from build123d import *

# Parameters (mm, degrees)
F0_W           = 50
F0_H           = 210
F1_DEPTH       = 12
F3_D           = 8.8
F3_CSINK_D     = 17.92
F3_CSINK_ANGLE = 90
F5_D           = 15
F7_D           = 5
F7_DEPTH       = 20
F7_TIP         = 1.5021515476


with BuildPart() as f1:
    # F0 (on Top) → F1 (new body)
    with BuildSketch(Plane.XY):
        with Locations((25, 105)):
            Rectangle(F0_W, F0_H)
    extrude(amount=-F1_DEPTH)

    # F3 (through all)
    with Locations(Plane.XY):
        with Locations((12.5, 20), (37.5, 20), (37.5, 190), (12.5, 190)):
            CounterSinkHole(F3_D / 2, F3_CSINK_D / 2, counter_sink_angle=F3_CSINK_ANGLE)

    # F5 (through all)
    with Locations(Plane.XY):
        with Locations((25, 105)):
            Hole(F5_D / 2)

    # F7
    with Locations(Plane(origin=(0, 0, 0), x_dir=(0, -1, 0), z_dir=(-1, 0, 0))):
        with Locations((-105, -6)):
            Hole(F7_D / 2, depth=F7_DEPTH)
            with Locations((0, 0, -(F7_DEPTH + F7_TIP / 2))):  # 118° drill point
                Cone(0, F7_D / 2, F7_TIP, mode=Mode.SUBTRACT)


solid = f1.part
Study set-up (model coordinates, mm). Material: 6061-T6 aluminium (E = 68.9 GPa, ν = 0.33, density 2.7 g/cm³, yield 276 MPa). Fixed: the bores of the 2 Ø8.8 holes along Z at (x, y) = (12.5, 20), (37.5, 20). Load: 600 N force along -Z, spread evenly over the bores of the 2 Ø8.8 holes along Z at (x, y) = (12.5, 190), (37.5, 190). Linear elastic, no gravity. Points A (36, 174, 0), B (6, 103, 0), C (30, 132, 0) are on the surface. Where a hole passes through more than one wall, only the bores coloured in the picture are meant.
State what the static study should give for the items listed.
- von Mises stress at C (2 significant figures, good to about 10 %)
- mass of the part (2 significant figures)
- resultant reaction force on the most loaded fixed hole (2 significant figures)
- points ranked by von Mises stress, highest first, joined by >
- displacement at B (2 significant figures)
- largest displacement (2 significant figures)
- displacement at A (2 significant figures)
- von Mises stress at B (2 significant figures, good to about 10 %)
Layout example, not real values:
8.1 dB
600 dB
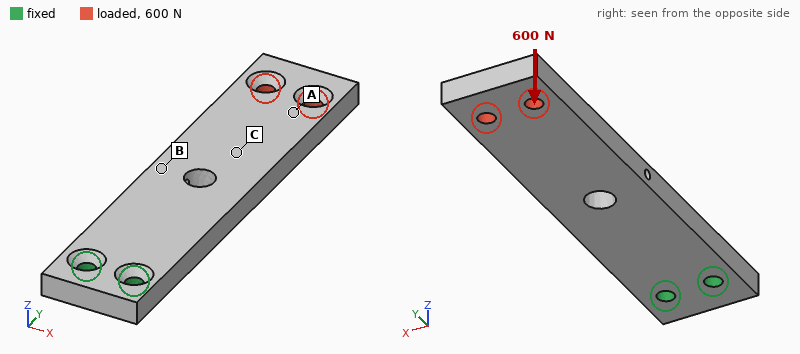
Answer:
29 MPa
320 g
470 N
B > C > A
0.67 mm
2.6 mm
1.9 mm
59 MPa
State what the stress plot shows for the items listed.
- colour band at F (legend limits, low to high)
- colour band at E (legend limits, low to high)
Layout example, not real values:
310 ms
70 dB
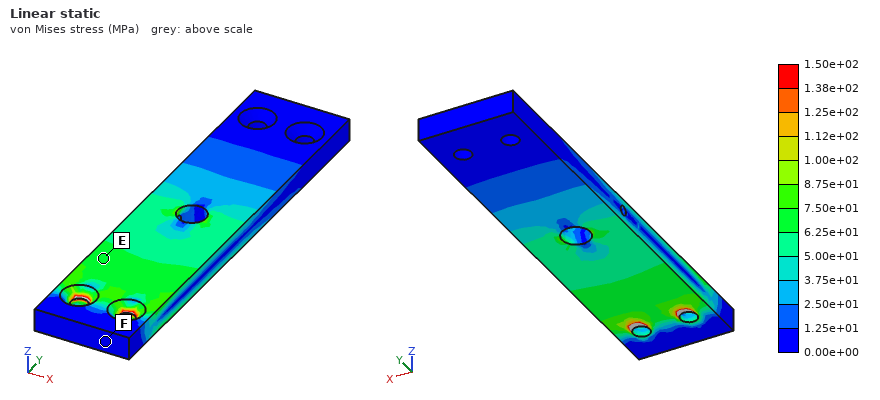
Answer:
0.00e+00 to 1.25e+01 MPa
6.25e+01 to 7.50e+01 MPa
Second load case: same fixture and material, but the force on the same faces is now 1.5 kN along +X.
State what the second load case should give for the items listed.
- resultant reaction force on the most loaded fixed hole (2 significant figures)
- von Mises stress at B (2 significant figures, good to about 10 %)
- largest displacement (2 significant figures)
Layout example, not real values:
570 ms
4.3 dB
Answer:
8.5 kN
25 MPa
0.42 mm
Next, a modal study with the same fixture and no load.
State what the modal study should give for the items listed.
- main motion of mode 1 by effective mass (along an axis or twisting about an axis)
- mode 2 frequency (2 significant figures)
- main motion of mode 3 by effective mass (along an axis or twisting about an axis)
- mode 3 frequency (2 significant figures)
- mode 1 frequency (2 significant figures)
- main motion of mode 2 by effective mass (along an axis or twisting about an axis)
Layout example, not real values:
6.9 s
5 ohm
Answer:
along Z
1000 Hz
along Z
1600 Hz
260 Hz
along X
